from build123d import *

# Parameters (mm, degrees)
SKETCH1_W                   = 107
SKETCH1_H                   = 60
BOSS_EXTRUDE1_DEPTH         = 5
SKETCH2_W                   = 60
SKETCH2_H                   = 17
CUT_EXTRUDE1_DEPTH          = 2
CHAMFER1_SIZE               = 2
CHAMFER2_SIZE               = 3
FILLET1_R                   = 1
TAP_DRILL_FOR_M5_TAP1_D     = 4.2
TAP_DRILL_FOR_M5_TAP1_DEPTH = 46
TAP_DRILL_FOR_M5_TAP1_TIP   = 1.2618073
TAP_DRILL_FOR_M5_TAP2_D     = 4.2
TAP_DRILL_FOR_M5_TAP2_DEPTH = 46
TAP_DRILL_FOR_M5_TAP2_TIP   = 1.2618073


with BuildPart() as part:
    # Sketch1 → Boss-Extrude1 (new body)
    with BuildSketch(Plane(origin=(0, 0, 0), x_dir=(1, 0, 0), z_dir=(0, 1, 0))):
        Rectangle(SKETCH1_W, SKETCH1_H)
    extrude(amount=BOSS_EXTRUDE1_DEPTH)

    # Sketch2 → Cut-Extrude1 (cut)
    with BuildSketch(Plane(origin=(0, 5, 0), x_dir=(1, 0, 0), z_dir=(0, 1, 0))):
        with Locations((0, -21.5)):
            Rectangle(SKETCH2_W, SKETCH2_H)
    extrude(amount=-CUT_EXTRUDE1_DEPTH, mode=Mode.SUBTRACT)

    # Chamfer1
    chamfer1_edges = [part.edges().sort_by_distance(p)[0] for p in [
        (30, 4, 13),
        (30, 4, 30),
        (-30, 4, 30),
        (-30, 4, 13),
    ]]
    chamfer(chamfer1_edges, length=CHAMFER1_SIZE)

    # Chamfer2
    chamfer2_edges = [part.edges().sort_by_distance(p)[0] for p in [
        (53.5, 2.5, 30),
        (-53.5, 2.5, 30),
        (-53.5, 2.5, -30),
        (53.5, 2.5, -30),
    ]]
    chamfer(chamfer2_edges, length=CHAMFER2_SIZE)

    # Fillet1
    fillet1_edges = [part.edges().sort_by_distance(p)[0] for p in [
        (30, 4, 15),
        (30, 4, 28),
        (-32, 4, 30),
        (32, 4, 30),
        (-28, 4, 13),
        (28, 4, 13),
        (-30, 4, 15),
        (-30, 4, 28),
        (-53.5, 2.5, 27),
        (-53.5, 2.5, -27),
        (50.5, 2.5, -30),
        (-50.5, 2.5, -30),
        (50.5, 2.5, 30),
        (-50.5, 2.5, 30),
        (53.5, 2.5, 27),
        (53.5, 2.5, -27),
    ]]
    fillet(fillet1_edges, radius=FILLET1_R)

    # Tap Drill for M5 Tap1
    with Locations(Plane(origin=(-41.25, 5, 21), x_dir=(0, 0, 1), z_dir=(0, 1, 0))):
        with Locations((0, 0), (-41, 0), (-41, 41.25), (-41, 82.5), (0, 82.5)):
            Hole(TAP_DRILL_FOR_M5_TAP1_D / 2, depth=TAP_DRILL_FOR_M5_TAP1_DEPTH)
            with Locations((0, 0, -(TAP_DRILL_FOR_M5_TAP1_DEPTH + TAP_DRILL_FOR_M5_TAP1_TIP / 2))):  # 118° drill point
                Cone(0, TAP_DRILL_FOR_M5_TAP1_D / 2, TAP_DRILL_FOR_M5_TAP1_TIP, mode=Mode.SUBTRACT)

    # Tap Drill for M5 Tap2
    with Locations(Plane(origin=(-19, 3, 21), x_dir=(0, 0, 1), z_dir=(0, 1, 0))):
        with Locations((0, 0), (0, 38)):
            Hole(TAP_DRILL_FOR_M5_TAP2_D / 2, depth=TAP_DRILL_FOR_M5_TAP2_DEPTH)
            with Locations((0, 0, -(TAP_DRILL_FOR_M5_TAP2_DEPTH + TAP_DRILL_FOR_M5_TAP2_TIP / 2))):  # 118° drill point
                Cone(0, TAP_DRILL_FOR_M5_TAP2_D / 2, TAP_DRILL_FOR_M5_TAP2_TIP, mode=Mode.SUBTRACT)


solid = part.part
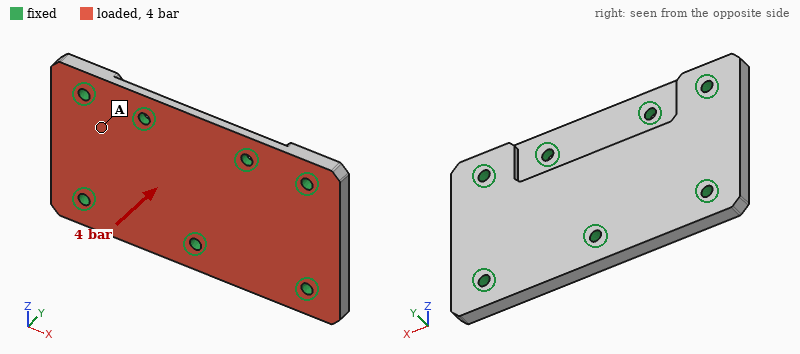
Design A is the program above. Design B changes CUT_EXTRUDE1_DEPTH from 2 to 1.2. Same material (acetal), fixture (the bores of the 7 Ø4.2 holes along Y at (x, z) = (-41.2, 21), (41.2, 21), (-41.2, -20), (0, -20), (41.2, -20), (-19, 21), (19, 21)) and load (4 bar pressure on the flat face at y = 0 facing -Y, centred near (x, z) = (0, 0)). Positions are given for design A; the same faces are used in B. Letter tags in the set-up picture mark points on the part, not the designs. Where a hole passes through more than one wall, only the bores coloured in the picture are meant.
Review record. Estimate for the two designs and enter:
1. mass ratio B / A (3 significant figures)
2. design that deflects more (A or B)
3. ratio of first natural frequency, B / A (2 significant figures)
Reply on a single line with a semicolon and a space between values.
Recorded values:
1.03; A; 1.1
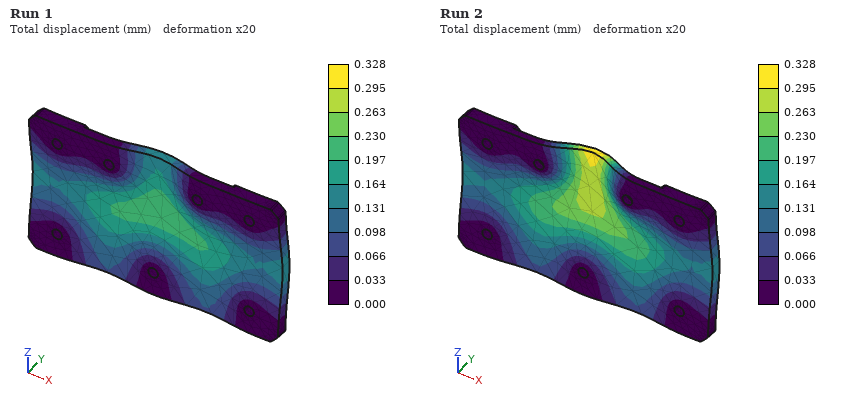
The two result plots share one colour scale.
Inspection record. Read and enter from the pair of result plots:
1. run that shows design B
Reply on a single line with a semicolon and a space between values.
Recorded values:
Run 1
